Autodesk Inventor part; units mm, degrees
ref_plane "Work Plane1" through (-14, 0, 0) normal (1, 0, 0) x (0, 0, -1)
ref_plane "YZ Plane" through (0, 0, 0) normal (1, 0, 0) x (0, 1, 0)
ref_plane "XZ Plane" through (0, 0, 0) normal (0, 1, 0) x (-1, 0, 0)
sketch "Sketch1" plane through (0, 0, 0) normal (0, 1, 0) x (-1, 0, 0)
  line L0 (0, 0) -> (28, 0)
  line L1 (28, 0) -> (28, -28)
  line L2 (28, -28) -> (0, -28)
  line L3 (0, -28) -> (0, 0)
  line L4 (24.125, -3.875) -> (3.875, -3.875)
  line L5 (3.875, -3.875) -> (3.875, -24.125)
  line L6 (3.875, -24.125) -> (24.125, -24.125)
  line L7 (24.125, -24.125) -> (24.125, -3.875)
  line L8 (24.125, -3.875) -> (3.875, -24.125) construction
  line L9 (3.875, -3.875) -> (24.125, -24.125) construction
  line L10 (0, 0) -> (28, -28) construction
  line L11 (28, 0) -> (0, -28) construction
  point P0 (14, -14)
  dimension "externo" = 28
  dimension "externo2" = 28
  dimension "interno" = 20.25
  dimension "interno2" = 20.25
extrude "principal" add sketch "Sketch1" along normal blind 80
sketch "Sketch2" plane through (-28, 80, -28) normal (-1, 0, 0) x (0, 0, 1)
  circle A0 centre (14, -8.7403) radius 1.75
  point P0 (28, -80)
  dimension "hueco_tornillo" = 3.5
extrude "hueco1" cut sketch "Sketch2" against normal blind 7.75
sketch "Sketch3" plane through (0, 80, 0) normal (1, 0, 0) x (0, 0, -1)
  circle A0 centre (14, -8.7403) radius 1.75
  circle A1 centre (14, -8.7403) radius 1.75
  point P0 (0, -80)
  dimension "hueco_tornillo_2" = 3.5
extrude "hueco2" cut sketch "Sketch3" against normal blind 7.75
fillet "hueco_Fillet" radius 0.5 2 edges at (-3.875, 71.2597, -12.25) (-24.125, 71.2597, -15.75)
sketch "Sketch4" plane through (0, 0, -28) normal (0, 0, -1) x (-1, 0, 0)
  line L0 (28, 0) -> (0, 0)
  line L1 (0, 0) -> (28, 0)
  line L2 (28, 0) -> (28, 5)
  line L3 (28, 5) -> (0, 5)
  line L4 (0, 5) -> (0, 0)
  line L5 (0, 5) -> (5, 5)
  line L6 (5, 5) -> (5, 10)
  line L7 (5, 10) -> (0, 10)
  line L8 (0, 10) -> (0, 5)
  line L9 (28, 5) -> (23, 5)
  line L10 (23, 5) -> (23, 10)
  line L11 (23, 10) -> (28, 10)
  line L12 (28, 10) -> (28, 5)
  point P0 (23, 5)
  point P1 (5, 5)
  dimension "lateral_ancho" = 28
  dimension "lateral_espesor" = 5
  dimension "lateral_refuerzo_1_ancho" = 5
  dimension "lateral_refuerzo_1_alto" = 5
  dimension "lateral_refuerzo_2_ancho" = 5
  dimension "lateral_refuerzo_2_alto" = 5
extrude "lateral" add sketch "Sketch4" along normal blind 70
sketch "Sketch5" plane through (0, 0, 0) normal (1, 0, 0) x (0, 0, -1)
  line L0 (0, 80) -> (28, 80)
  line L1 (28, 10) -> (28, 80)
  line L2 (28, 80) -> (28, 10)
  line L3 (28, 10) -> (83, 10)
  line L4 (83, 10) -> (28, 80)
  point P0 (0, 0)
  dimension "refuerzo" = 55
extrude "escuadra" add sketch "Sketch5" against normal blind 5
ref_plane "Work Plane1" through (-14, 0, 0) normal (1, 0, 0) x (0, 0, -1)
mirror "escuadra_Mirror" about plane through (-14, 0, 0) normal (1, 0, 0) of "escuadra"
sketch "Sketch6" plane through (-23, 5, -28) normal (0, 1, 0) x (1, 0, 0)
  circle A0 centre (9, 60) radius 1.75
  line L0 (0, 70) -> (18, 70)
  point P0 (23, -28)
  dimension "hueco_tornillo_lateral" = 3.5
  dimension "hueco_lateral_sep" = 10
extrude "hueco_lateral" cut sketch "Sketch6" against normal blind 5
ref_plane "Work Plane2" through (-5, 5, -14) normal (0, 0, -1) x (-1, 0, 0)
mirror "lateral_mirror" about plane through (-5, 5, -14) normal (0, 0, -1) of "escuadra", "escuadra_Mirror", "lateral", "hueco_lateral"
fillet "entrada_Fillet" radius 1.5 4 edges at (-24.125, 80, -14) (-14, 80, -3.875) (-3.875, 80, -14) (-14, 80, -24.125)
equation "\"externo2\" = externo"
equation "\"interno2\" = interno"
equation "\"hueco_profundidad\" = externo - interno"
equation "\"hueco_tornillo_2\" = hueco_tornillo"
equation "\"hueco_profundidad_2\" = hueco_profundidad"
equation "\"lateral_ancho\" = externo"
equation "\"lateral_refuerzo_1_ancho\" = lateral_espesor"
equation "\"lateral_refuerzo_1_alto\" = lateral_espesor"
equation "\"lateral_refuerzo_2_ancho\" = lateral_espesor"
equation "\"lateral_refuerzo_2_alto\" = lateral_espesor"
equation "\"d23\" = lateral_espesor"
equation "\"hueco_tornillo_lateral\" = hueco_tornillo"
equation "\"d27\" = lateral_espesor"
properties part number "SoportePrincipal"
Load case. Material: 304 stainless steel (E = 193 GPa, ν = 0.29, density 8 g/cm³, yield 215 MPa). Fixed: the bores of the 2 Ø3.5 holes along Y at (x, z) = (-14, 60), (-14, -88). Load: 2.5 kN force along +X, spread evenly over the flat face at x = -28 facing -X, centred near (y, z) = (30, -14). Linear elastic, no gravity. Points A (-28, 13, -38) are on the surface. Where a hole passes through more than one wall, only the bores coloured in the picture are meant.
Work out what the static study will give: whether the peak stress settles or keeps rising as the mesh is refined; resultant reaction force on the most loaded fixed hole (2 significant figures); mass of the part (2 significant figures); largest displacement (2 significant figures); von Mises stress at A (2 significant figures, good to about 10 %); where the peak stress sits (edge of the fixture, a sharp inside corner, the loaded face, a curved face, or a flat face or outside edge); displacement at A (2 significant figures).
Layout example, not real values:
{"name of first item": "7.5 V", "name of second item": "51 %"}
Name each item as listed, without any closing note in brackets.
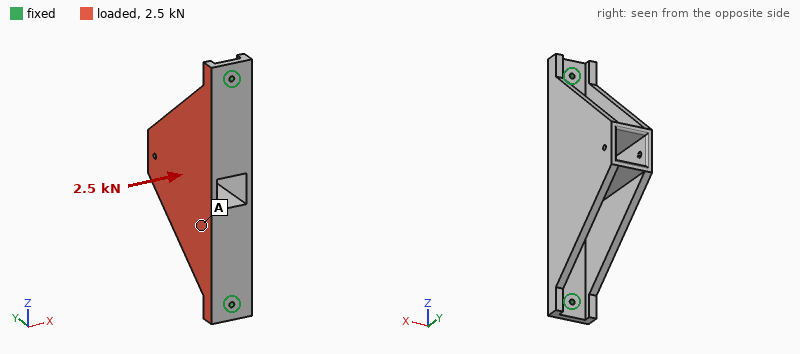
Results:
{"whether the peak stress settles or keeps rising as the mesh is refined": "keeps rising", "resultant reaction force on the most loaded fixed hole": "1.3 kN", "mass of the part": "760 g", "largest displacement": "0.47 mm", "von Mises stress at A": "29 MPa", "where the peak stress sits": "edge of the fixture", "displacement at A": "0.12 mm"}
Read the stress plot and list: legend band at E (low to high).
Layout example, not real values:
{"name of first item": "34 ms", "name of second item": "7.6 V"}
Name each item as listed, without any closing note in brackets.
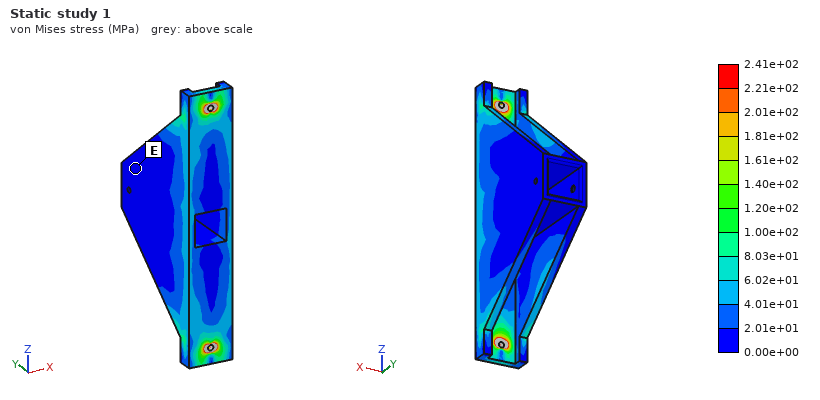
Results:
{"legend band at E": "0.00e+00 to 2.01e+01 MPa"}
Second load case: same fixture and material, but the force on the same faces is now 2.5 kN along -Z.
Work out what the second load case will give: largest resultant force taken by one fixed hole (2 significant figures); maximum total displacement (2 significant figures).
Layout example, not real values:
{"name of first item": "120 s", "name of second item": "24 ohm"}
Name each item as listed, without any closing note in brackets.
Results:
{"largest resultant force taken by one fixed hole": "1.4 kN", "maximum total displacement": "7.6 µm"}
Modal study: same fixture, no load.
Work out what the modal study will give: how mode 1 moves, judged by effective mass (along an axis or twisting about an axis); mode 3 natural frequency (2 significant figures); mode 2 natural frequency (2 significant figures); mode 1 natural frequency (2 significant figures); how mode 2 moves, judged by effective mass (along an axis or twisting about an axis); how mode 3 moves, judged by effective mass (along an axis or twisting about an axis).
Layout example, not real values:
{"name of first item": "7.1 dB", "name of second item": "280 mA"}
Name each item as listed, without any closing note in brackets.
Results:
{"how mode 1 moves, judged by effective mass": "along X", "mode 3 natural frequency": "3400 Hz", "mode 2 natural frequency": "2800 Hz", "mode 1 natural frequency": "570 Hz", "how mode 2 moves, judged by effective mass": "along Y", "how mode 3 moves, judged by effective mass": "along X"}
